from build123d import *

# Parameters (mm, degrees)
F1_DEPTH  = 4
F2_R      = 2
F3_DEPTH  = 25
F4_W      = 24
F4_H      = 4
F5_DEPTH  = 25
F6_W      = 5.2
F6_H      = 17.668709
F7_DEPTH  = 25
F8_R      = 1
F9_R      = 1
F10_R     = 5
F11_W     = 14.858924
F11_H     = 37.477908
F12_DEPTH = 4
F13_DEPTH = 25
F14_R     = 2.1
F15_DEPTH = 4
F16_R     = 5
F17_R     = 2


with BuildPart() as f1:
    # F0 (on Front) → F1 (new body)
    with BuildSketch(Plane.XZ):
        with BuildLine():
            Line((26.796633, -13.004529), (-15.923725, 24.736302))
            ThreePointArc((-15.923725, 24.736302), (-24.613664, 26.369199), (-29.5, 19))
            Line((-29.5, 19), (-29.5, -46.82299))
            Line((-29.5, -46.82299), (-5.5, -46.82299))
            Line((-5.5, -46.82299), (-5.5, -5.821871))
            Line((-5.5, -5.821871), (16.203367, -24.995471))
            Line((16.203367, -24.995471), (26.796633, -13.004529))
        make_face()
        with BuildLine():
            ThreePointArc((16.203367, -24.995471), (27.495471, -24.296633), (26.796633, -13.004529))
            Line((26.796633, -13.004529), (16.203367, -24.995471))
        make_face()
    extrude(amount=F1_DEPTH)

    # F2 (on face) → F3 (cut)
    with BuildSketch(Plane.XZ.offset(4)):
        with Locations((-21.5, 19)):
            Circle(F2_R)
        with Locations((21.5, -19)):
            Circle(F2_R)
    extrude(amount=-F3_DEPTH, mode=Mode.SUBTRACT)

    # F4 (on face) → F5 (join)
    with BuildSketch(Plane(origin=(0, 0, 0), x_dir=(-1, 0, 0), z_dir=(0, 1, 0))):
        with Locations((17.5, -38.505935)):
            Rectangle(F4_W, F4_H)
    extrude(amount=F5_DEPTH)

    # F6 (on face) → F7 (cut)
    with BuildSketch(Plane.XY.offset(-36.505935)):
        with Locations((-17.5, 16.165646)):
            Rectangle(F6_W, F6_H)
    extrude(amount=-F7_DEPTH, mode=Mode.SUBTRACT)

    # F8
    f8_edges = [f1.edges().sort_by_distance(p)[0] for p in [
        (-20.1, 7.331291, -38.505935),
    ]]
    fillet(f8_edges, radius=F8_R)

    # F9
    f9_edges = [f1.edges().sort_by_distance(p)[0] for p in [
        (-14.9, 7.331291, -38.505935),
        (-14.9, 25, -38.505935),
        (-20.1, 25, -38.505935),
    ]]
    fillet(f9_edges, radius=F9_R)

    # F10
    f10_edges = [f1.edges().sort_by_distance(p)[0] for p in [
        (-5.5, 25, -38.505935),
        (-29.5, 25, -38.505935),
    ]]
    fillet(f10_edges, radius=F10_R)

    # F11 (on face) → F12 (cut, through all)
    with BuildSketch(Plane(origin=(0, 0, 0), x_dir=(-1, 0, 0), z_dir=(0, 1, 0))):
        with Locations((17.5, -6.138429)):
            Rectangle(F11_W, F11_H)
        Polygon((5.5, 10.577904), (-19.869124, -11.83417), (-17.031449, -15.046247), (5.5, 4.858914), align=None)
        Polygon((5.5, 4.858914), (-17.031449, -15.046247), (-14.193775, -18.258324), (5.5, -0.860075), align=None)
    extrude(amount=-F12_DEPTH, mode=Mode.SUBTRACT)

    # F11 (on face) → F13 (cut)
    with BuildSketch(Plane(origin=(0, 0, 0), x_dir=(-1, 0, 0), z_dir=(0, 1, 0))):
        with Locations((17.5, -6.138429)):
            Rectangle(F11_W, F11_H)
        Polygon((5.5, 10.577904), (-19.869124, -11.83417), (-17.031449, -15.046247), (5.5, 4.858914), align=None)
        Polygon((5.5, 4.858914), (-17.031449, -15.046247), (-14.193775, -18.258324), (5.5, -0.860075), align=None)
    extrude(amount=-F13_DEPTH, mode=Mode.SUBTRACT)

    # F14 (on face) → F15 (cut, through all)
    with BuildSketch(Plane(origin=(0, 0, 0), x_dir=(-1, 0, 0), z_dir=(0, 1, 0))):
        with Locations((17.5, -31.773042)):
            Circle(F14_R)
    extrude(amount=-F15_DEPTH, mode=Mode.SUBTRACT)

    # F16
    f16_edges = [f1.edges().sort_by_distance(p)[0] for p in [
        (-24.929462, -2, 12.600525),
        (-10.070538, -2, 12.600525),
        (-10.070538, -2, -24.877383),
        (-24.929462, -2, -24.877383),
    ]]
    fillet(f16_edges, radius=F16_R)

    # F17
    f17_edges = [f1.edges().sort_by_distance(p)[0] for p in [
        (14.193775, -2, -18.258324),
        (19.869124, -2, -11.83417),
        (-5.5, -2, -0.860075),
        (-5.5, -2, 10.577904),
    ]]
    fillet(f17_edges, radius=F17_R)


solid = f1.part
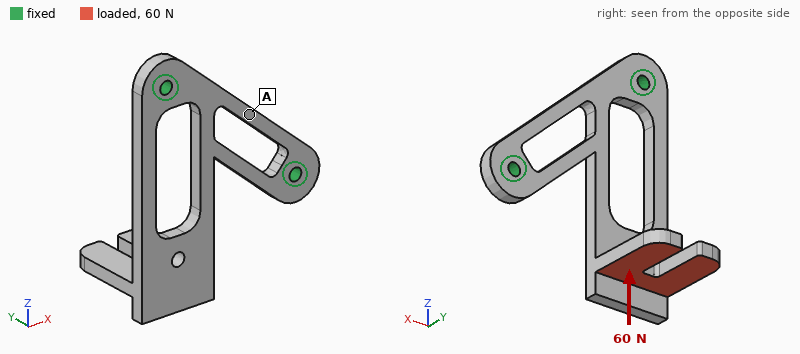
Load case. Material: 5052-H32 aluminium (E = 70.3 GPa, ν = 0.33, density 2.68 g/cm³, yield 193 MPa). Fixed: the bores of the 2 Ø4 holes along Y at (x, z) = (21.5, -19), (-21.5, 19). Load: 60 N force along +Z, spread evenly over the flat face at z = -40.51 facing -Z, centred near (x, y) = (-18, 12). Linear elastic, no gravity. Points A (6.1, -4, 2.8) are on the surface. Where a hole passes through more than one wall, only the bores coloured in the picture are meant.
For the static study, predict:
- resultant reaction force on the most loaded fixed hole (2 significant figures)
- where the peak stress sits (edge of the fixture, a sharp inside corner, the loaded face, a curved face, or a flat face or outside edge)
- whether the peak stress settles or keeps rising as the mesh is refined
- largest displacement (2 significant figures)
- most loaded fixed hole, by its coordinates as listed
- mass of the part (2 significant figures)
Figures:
53 N
a sharp inside corner
keeps rising
0.39 mm
(-21.5, 19)
22 g
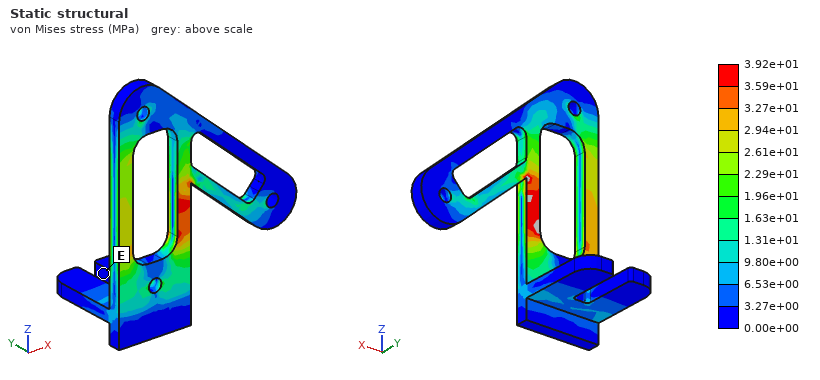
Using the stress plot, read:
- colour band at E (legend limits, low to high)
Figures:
0.00e+00 to 3.27e+00 MPa
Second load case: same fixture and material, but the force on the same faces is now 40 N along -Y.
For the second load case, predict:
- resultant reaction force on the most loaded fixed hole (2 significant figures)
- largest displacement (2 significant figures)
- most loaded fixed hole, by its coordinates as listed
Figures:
28 N
0.65 mm
(21.5, -19)
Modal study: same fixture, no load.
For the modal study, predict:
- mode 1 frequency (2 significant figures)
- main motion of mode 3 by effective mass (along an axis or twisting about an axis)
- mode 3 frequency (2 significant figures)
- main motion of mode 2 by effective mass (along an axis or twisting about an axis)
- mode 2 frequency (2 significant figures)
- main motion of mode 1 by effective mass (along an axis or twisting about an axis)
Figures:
440 Hz
along X
2000 Hz
along X
1200 Hz
along Y
